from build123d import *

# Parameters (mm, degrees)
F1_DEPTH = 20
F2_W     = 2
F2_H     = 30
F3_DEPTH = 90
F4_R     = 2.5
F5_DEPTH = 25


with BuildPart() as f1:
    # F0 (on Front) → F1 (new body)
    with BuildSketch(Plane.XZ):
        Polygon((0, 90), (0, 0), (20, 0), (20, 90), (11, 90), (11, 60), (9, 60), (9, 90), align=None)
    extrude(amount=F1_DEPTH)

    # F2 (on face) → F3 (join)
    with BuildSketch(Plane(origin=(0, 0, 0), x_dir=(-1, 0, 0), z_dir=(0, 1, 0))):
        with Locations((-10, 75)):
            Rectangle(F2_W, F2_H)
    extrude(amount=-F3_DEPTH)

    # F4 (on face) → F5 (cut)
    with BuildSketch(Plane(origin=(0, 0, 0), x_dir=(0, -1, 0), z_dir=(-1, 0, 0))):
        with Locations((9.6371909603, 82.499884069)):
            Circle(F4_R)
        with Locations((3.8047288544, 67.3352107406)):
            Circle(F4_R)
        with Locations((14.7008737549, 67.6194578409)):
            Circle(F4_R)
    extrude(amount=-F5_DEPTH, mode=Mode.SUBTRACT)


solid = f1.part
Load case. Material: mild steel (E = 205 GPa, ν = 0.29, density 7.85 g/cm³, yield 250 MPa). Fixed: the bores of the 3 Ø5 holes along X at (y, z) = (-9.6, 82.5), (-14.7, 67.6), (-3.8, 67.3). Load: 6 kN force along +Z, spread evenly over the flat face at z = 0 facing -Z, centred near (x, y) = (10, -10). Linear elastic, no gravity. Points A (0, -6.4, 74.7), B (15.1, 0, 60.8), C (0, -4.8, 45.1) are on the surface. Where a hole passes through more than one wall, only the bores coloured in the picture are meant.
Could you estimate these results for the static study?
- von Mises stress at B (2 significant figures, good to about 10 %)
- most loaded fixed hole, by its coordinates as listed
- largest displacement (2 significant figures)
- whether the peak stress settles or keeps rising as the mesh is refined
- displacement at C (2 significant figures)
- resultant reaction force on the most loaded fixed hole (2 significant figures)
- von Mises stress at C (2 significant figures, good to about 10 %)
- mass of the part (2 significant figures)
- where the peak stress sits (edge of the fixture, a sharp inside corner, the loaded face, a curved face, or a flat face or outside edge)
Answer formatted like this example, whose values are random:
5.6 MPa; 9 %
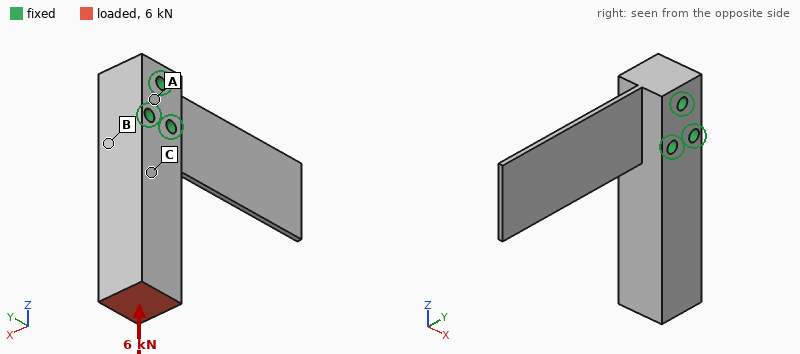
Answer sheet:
13 MPa; (-14.7, 67.6); 4.9 µm; keeps rising; 1.5 µm; 3.2 kN; 15 MPa; 310 g; edge of the fixture
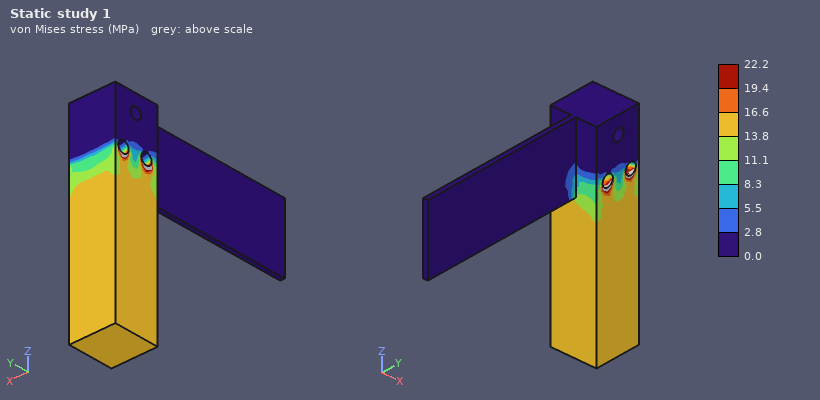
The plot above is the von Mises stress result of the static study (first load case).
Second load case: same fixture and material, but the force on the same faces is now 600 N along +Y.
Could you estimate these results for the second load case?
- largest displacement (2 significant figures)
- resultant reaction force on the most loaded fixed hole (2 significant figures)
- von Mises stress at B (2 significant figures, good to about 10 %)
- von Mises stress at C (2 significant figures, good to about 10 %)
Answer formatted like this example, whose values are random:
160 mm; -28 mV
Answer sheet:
23 µm; 2.9 kN; 25 MPa; 11 MPa
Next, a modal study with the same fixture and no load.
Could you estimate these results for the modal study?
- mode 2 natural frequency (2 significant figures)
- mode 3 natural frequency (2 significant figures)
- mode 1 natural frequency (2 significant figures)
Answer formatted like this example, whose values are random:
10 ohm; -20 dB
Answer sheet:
1700 Hz; 2100 Hz; 340 Hz
